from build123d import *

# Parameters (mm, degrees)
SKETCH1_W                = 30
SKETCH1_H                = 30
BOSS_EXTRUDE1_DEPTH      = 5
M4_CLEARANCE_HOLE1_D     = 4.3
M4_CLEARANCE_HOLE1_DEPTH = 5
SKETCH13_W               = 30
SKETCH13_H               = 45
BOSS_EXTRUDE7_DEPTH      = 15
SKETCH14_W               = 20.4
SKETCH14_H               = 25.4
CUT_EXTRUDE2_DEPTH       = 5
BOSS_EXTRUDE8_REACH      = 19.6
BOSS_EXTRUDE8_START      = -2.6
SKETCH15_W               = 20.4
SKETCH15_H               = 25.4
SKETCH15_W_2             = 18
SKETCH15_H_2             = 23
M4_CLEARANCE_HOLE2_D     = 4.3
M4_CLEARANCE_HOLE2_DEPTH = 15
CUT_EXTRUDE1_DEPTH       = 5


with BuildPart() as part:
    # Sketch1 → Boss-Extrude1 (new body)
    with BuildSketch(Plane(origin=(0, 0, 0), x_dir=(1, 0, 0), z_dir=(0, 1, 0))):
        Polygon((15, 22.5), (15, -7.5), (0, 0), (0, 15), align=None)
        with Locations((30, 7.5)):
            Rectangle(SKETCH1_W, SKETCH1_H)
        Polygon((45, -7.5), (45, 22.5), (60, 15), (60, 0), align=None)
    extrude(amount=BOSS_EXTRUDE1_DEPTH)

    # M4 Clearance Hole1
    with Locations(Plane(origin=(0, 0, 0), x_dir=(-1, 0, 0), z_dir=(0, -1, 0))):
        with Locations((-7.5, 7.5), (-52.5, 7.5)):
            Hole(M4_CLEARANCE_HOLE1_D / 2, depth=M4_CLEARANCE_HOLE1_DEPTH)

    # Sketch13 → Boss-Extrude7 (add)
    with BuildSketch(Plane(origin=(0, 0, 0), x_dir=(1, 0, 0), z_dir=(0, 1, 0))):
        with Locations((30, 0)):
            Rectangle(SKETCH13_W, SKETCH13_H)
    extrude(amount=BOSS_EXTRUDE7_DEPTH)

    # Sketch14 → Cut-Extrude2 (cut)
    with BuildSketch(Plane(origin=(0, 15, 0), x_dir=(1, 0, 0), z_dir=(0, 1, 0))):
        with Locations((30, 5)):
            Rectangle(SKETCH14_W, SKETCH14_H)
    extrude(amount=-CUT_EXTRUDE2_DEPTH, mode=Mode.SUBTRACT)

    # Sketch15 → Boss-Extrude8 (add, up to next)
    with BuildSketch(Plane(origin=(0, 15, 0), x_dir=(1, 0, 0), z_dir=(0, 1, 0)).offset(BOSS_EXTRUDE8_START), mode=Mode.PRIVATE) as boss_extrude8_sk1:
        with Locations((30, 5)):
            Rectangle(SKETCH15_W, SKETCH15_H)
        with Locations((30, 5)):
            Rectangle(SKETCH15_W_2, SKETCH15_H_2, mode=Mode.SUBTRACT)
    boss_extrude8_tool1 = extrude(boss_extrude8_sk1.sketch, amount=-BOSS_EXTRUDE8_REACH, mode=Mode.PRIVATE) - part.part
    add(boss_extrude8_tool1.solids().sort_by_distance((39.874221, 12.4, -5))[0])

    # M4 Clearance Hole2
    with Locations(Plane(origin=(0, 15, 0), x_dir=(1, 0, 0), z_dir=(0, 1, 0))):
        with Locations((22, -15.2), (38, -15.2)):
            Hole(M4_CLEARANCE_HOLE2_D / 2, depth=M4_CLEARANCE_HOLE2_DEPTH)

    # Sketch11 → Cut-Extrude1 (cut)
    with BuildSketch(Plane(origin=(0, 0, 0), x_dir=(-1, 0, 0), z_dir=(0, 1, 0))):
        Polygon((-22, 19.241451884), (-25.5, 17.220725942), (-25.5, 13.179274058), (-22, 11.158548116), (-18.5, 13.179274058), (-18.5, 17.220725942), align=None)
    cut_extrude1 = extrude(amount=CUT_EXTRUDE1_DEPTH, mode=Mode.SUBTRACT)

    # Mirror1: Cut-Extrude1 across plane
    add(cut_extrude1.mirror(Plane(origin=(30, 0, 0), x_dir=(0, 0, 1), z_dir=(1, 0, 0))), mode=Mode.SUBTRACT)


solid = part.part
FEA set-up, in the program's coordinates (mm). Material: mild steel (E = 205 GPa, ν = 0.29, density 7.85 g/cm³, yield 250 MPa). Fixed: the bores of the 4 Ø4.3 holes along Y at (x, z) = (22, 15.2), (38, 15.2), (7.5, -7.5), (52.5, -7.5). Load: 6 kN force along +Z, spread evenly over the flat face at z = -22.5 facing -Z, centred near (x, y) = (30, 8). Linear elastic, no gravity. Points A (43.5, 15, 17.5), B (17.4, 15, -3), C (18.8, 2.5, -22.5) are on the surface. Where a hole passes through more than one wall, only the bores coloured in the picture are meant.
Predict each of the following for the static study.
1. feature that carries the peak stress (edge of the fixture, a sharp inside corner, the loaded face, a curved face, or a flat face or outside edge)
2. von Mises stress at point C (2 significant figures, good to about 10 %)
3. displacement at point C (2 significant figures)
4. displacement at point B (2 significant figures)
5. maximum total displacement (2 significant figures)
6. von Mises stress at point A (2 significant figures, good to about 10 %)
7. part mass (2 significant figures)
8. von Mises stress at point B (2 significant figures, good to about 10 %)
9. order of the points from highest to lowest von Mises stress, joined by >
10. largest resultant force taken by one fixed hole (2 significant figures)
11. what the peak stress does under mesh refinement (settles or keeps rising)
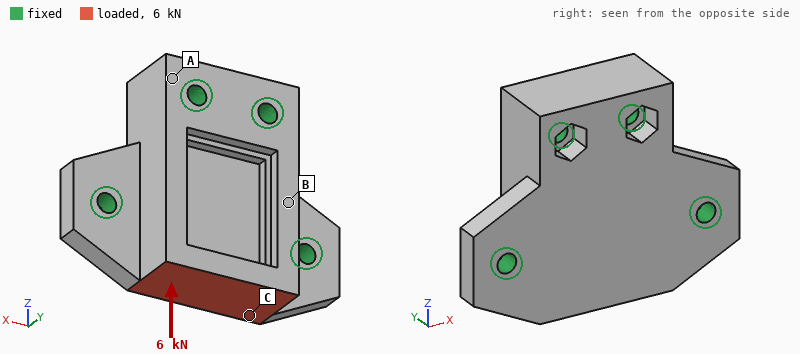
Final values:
edge of the fixture
13 MPa
3.9 µm
2.3 µm
8.6 µm
6.1 MPa
160 g
30 MPa
B > C > A
2.2 kN
keeps rising
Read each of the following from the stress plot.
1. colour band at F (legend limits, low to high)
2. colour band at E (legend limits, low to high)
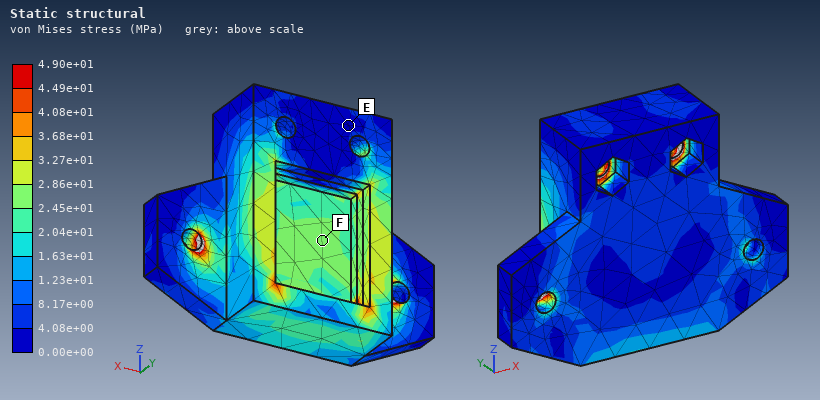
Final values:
2.45e+01 to 2.86e+01 MPa
0.00e+00 to 4.08e+00 MPa
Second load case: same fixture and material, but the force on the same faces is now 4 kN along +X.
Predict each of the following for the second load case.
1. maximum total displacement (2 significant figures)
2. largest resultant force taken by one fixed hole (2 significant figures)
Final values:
5.7 µm
2.2 kN
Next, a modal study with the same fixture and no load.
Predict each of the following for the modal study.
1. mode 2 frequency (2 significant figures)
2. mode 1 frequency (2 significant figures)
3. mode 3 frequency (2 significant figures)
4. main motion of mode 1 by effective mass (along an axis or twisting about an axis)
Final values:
23 kHz
12 kHz
28 kHz
along Y
